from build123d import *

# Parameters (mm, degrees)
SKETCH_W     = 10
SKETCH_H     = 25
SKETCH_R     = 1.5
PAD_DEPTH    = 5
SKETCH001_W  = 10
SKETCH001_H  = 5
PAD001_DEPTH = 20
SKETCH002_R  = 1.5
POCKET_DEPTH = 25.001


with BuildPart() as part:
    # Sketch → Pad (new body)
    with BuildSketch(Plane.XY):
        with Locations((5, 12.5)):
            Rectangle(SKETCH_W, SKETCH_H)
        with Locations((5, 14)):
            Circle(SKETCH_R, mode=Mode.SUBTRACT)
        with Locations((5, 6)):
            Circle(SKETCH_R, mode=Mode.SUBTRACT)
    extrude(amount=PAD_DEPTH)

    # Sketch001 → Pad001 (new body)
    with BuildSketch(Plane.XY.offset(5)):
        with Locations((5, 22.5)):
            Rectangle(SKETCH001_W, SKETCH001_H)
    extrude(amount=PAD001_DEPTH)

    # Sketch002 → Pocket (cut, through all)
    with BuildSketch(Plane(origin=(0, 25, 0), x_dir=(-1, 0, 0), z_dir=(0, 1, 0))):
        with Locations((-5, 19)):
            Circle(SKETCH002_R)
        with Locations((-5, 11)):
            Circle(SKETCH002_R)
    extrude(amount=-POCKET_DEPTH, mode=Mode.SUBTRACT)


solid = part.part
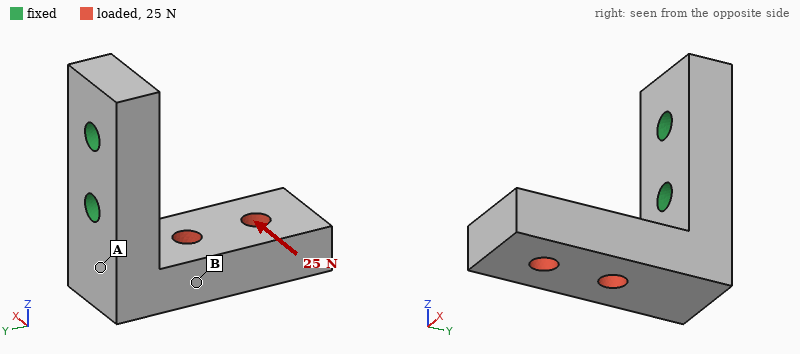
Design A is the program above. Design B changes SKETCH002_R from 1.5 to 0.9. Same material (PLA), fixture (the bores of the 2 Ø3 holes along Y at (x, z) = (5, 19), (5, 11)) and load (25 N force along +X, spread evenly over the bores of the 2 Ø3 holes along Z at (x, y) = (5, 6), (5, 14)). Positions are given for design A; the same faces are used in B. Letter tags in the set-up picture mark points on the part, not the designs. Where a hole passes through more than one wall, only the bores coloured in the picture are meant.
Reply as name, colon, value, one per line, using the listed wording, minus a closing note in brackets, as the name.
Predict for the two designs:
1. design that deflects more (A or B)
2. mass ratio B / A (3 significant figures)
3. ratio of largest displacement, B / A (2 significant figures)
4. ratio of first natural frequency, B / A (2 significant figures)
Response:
design that deflects more: B
mass ratio B / A: 1.02
ratio of largest displacement, B / A: 1.2
ratio of first natural frequency, B / A: 0.96
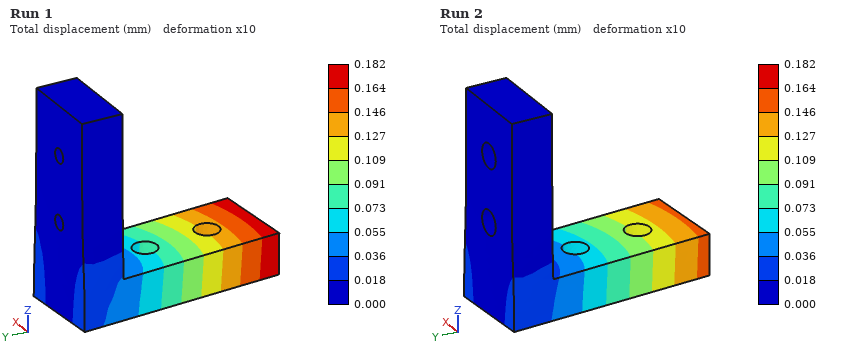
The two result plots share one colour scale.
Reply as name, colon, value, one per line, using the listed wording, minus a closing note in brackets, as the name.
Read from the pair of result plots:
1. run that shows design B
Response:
run that shows design B: Run 1
